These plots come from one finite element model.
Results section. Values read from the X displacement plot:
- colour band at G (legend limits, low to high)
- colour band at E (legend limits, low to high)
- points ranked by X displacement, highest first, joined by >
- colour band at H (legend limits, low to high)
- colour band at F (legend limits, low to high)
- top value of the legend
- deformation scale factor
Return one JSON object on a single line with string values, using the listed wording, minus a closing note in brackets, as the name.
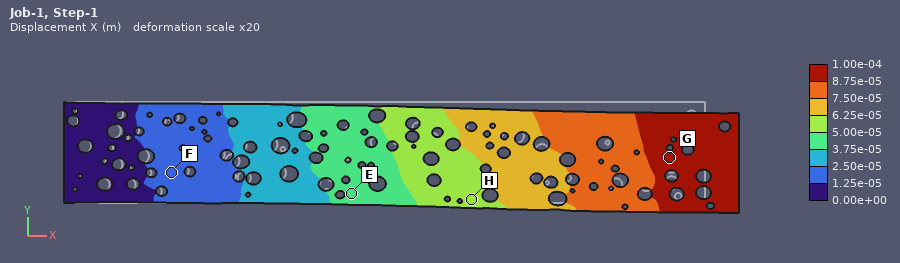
{"colour band at G": "8.75e-05 to 1.00e-04 m", "colour band at E": "3.75e-05 to 5.00e-05 m", "points ranked by X displacement, highest first, joined by >": "G > H > E > F", "colour band at H": "5.00e-05 to 6.25e-05 m", "colour band at F": "1.25e-05 to 2.50e-05 m", "top value of the legend": "1.00e-04 m", "deformation scale factor": "20"}
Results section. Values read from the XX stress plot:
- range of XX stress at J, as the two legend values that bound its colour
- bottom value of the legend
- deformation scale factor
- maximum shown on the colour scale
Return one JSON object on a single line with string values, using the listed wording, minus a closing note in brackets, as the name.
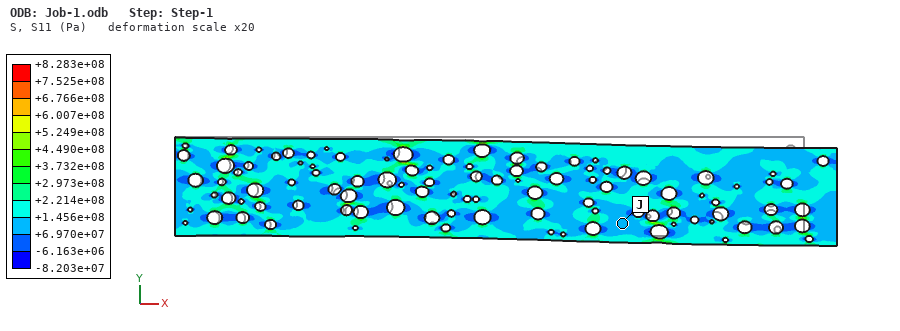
{"range of XX stress at J, as the two legend values that bound its colour": "+6.970e+07 to +1.456e+08 Pa", "bottom value of the legend": "-8.203e+07 Pa", "deformation scale factor": "20", "maximum shown on the colour scale": "+8.283e+08 Pa"}
